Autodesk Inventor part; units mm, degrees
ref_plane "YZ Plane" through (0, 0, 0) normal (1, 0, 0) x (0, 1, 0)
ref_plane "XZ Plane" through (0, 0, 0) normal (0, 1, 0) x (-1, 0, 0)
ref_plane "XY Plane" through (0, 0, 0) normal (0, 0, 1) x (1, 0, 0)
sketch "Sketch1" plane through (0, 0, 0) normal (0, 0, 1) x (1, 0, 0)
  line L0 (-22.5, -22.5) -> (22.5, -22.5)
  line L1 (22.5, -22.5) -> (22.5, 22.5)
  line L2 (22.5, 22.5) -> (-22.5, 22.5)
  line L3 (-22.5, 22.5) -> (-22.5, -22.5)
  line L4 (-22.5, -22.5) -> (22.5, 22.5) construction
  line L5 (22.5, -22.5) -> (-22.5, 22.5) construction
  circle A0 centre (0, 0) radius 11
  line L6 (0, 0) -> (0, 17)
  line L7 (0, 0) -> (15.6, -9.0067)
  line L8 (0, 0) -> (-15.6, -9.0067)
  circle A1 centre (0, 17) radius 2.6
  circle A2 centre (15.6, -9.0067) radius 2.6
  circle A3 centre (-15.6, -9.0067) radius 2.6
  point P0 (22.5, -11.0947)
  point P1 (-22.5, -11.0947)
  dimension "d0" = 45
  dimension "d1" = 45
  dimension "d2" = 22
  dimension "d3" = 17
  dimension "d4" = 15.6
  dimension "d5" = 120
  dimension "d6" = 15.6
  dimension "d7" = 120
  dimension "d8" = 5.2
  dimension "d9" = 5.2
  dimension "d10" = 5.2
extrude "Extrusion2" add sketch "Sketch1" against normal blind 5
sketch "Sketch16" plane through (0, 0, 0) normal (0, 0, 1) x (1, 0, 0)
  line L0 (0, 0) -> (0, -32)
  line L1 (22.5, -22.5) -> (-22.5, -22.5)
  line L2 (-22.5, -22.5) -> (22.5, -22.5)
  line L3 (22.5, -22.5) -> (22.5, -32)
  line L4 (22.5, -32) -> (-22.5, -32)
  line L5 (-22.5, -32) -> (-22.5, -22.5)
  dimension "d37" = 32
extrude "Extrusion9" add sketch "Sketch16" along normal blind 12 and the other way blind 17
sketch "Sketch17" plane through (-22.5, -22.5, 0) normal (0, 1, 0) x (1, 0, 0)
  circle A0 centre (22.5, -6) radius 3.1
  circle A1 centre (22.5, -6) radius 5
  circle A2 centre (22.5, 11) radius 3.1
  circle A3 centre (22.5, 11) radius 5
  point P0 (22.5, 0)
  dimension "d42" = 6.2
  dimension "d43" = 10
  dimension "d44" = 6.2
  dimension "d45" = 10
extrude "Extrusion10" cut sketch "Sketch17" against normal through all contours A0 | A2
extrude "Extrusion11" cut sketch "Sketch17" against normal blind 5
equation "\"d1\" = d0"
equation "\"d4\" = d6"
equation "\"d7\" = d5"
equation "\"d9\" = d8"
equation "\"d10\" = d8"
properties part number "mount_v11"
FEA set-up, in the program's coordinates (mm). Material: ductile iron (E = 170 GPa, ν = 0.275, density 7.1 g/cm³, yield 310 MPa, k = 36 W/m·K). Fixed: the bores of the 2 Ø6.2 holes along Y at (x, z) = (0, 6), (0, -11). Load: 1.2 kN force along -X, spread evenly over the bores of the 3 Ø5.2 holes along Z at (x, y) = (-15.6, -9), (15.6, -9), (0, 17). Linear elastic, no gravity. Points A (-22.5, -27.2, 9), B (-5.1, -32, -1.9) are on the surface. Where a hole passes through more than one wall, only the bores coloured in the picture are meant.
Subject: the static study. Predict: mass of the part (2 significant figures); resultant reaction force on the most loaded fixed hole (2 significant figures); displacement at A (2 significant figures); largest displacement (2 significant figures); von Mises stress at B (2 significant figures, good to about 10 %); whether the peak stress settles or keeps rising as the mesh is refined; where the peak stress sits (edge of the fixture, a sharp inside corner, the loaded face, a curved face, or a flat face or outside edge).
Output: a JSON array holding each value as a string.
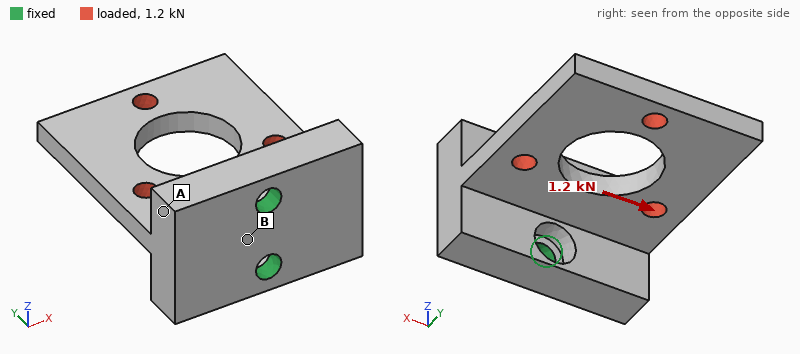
["140 g", "600 N", "22 µm", "66 µm", "31 MPa", "keeps rising", "edge of the fixture"]
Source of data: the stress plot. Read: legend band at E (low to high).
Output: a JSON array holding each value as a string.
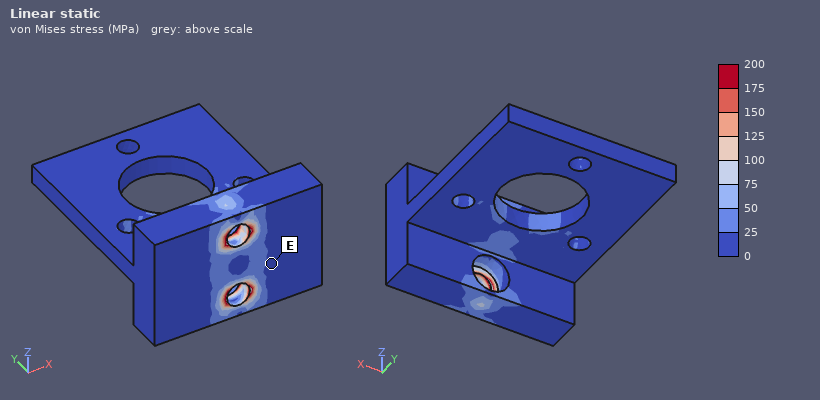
["0 to 25 MPa"]
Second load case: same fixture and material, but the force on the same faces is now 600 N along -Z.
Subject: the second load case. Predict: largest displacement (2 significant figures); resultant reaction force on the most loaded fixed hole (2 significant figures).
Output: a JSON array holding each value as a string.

["0.14 mm", "1.0 kN"]
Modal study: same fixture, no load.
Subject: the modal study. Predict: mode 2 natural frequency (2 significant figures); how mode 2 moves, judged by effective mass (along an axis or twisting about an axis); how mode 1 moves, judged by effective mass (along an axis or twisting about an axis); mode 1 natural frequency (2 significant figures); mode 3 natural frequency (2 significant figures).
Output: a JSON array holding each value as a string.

["3000 Hz", "along X", "along Z", "1600 Hz", "3600 Hz"]
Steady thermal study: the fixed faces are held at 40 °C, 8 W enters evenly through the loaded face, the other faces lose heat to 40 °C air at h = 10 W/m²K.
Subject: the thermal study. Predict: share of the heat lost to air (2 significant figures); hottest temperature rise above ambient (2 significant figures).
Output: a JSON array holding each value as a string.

["16 %", "41 K"]
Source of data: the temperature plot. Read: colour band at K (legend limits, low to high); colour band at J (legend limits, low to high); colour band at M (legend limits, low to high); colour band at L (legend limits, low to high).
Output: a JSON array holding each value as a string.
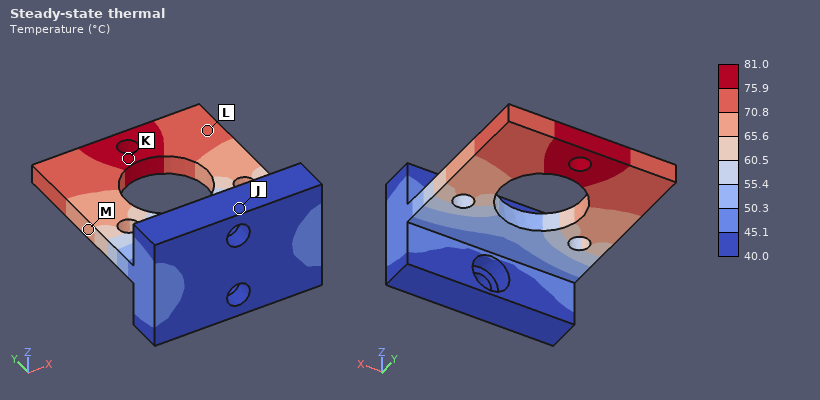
["75.9 to 81.0 °C", "40.0 to 45.1 °C", "65.6 to 70.8 °C", "70.8 to 75.9 °C"]
